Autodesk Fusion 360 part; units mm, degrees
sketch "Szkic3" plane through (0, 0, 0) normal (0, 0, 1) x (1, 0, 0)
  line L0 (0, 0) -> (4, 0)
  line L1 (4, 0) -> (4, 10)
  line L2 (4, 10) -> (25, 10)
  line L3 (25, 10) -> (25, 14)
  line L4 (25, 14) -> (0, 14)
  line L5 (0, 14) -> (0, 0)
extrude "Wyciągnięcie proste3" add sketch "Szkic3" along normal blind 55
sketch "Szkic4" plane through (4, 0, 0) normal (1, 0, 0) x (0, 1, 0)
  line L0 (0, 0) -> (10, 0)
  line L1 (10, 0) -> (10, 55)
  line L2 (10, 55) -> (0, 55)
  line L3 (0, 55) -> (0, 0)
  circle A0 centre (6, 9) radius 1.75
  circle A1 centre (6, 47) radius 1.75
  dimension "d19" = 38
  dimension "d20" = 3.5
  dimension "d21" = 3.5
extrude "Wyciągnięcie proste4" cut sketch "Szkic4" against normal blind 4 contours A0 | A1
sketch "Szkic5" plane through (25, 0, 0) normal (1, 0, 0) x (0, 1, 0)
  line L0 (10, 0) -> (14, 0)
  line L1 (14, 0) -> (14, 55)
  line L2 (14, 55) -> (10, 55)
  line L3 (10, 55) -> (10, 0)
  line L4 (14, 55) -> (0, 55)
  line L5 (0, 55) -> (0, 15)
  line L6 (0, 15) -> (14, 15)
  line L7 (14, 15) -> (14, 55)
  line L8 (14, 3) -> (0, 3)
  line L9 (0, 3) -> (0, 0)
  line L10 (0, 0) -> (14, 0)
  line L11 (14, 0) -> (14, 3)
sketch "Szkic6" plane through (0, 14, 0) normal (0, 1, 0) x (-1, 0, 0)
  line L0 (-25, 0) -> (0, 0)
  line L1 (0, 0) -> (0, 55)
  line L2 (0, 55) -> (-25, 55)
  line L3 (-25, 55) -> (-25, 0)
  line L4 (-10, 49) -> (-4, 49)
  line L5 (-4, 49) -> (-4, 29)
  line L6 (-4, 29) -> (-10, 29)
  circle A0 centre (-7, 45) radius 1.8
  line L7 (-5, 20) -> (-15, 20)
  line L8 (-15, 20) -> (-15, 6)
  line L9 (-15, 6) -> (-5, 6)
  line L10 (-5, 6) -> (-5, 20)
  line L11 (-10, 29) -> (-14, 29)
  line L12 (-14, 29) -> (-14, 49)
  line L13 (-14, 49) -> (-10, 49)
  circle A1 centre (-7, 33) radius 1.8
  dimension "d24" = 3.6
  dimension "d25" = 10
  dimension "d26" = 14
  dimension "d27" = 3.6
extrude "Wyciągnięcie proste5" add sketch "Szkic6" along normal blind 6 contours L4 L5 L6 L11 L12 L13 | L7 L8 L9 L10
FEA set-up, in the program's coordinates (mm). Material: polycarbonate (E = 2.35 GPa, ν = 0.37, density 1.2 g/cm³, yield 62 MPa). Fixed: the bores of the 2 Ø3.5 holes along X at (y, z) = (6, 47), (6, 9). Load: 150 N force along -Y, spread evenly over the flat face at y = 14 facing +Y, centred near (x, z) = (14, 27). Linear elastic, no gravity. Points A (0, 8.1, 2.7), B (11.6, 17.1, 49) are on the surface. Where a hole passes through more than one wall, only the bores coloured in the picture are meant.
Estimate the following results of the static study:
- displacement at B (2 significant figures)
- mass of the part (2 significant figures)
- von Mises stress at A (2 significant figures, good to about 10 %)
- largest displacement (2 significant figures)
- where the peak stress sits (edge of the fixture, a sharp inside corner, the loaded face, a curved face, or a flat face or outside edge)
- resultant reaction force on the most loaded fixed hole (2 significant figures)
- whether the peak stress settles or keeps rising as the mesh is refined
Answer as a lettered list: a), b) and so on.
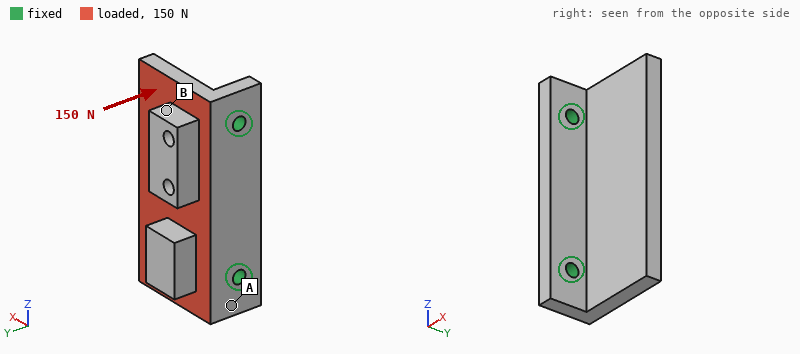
a) 0.32 mm
b) 11 g
c) 9.1 MPa
d) 0.70 mm
e) edge of the fixture
f) 79 N
g) keeps rising
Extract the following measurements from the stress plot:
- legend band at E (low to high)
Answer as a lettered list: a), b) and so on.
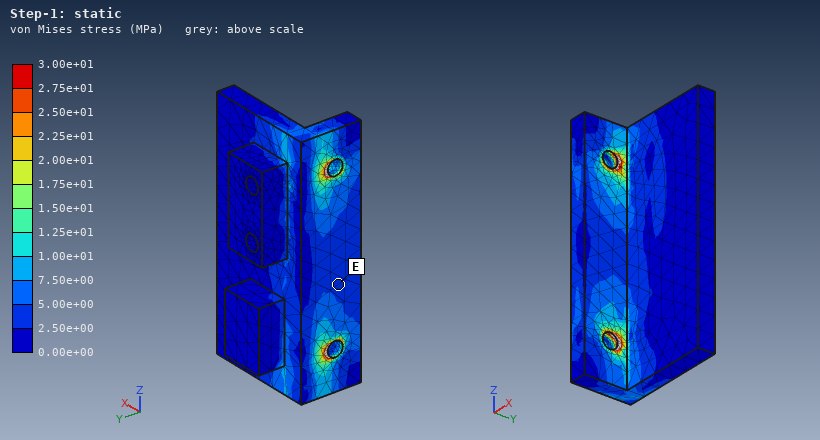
a) 2.50e+00 to 5.00e+00 MPa
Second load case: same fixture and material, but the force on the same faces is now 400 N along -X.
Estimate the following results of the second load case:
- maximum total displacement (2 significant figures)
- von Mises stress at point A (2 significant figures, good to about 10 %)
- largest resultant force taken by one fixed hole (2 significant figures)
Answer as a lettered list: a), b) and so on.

a) 0.74 mm
b) 11 MPa
c) 210 N
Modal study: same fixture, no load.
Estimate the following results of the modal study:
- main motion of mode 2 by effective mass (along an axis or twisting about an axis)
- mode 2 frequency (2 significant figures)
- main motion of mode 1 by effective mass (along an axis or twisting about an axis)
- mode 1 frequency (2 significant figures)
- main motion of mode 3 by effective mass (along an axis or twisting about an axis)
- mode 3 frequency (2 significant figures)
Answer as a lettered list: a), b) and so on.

a) twisting about X
b) 2100 Hz
c) along Y
d) 1000 Hz
e) along X
f) 3800 Hz
